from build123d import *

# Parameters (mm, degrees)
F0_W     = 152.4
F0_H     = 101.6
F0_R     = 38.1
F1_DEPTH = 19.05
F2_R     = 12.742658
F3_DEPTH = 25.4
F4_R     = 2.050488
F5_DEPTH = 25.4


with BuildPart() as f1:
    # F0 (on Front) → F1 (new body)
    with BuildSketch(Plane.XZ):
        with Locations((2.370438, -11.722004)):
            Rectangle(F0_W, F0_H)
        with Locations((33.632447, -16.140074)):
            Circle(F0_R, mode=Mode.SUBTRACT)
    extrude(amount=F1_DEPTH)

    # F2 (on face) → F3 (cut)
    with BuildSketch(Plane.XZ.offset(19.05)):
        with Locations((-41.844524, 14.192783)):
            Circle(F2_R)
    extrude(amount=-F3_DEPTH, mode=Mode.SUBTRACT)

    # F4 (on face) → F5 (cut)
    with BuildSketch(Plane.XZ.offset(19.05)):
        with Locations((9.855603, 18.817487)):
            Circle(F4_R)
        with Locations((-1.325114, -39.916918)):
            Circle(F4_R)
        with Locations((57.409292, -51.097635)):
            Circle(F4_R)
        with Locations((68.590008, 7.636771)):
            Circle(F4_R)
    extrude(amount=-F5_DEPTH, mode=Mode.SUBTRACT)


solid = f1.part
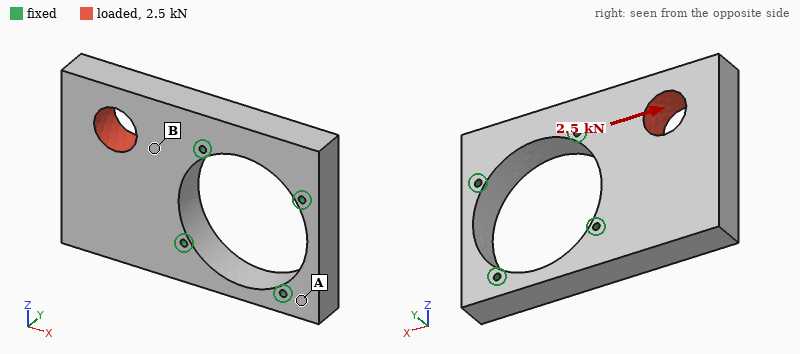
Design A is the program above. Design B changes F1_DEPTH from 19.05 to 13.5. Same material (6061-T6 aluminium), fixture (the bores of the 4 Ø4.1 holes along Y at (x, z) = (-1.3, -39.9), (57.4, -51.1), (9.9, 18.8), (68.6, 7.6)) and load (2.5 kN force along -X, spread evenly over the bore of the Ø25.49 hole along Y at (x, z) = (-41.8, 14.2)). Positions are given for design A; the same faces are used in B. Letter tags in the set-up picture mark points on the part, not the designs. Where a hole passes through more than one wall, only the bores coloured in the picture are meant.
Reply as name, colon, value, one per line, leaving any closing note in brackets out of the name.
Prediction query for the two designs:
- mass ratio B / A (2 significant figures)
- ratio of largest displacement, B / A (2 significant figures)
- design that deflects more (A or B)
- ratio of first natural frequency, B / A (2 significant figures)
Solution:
mass ratio B / A: 0.71
ratio of largest displacement, B / A: 1.4
design that deflects more: B
ratio of first natural frequency, B / A: 0.74
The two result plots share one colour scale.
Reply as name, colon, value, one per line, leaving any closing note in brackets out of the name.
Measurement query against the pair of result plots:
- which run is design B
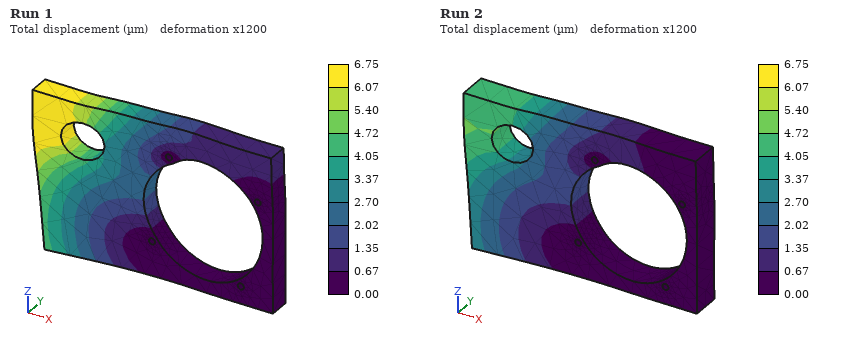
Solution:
which run is design B: Run 1
